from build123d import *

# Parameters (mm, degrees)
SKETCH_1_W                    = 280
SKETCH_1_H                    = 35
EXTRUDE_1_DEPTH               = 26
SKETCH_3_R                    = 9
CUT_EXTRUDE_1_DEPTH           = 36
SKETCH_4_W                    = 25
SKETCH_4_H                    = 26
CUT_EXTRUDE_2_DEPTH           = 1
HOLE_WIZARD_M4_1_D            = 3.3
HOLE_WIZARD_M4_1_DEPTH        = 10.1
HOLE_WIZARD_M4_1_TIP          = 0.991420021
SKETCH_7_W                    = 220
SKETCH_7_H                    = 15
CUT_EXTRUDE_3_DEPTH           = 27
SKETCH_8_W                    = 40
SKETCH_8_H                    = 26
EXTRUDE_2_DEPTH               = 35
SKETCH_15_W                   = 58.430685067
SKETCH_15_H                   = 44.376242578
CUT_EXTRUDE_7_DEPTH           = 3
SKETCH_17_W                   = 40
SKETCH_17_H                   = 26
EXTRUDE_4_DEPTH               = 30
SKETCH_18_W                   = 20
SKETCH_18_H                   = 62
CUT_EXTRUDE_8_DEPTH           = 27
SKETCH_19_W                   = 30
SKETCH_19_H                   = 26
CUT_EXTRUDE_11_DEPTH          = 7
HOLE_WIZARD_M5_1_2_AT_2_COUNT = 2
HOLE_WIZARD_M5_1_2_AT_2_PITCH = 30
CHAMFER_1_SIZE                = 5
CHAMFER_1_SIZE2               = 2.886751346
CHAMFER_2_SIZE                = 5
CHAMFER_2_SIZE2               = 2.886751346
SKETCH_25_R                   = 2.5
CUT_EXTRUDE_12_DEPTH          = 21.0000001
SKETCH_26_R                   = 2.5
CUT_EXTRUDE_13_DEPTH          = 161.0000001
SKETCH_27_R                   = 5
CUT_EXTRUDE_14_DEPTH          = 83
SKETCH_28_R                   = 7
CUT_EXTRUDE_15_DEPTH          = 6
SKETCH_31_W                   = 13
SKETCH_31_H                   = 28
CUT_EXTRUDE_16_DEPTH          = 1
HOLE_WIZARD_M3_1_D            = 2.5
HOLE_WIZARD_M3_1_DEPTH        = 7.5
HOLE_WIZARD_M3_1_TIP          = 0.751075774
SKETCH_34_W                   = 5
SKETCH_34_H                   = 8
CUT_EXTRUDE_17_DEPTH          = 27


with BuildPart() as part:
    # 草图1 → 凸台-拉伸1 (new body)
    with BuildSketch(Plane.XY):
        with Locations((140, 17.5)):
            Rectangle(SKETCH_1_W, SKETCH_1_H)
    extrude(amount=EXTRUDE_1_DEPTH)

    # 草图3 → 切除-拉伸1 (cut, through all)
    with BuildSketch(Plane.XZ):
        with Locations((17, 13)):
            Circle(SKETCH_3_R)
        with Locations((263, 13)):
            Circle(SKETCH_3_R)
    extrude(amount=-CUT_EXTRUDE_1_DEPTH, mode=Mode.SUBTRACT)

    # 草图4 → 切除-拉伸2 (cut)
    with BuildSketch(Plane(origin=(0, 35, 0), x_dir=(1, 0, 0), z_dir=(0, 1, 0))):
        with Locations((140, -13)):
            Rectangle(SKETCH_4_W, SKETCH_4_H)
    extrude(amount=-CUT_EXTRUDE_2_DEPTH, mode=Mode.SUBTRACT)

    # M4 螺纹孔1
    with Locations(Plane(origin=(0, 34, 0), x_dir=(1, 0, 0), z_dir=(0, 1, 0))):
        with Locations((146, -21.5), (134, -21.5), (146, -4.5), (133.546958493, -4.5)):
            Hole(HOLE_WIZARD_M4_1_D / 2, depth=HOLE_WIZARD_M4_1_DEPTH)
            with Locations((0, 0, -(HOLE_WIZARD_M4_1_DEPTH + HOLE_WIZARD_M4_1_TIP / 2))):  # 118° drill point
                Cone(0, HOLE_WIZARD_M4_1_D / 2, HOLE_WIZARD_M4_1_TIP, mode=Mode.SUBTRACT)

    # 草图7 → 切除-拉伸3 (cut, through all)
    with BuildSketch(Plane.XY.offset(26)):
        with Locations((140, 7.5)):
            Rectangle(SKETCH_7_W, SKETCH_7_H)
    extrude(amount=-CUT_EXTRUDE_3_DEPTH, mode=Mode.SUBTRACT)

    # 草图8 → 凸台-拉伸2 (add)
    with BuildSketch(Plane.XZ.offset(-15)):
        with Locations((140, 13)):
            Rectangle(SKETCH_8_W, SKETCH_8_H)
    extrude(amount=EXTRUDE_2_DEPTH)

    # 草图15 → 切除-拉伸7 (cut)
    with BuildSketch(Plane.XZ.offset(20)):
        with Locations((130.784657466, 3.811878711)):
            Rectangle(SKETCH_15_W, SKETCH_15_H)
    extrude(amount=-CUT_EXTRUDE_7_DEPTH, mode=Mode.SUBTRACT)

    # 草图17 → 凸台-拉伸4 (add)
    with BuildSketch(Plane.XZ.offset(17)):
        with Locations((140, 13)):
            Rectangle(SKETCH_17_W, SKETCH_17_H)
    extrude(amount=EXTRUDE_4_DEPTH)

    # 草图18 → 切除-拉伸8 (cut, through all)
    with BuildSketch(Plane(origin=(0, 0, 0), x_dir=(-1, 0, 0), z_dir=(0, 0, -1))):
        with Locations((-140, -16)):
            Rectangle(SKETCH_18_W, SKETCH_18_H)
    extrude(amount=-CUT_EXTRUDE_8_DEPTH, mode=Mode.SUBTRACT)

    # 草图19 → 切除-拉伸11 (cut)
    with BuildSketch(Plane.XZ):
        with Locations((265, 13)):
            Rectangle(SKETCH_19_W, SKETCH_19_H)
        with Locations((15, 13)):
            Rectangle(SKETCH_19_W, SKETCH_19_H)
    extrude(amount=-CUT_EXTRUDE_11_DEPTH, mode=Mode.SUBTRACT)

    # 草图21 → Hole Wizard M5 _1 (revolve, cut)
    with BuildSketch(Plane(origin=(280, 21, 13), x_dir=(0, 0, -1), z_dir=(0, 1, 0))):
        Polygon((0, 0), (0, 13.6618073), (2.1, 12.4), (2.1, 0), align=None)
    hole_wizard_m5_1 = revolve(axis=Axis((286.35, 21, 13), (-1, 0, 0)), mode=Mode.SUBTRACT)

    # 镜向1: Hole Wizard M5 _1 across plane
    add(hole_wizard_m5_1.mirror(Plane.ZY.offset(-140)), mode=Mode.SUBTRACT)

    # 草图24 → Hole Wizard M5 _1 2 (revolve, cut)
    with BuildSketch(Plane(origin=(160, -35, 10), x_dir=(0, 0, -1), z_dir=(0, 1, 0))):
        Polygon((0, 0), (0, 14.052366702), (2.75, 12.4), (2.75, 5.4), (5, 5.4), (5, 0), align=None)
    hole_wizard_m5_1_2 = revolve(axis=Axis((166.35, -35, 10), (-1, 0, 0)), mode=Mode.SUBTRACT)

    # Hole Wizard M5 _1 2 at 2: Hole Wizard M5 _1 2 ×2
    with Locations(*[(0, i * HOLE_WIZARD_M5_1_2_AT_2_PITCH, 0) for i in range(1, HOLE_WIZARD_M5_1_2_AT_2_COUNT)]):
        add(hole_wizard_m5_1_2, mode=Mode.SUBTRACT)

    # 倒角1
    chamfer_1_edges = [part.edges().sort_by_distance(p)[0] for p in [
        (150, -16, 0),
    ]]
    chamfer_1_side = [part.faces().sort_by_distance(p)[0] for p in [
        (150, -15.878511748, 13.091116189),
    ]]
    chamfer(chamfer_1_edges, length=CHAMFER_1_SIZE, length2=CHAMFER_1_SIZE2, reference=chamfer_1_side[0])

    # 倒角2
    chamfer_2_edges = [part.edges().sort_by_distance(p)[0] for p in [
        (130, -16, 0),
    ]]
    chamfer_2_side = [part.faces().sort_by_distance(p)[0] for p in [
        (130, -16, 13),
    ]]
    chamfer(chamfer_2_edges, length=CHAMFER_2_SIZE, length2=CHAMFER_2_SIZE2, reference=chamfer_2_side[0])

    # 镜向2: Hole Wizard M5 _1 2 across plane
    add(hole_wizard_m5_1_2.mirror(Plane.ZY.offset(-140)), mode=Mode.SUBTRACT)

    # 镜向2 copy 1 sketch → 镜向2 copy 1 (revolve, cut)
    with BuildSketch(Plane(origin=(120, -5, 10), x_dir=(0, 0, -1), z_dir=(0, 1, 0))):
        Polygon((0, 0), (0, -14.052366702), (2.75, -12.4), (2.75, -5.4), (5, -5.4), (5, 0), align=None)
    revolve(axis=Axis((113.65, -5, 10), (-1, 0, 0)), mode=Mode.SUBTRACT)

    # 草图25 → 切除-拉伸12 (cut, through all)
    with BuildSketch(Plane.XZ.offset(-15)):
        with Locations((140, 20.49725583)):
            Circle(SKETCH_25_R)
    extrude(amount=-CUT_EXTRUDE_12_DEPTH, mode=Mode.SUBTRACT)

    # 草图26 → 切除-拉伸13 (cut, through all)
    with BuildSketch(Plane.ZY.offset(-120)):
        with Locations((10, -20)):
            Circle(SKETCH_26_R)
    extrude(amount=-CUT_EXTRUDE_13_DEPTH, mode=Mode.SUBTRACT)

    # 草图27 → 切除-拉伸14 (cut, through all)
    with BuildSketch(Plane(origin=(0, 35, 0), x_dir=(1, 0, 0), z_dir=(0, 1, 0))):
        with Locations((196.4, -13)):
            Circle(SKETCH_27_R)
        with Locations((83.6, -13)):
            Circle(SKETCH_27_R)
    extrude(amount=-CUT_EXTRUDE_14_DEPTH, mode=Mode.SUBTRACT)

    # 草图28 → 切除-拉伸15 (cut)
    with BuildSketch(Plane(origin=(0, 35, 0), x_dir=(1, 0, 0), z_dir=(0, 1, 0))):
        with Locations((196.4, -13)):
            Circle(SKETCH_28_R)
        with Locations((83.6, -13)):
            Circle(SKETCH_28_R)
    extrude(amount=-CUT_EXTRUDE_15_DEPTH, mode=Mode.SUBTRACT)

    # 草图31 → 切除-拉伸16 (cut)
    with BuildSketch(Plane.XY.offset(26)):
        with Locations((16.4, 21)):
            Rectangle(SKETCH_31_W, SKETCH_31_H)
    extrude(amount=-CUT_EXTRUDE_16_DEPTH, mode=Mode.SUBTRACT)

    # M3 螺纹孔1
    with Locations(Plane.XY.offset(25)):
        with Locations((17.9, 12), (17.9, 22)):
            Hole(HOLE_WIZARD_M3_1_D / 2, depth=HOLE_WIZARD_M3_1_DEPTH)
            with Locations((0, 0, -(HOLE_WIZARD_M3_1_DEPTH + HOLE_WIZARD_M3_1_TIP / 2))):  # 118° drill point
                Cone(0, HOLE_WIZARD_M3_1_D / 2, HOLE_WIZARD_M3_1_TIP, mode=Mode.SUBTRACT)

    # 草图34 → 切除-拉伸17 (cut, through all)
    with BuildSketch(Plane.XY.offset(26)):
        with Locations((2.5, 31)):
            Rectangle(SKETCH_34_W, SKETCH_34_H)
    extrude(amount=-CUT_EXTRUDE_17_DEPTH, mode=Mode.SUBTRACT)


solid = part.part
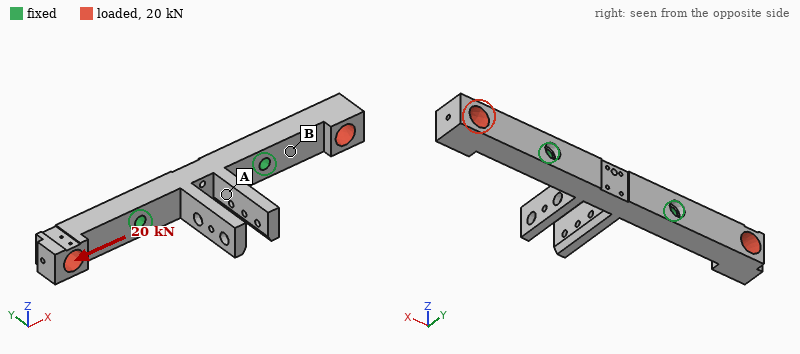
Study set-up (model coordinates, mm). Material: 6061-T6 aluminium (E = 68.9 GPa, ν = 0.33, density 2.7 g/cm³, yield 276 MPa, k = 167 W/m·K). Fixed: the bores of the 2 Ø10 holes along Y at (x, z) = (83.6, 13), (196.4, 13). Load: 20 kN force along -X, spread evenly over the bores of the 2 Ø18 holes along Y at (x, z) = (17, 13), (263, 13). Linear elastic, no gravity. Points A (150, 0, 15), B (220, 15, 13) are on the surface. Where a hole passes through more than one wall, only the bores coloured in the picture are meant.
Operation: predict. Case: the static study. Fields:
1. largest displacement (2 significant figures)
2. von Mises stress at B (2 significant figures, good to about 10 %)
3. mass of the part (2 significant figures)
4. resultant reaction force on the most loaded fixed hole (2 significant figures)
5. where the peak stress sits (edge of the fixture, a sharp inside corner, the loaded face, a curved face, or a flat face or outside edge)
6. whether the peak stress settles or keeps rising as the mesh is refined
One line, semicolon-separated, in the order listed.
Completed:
0.12 mm; 44 MPa; 450 g; 10 kN; a sharp inside corner; keeps rising
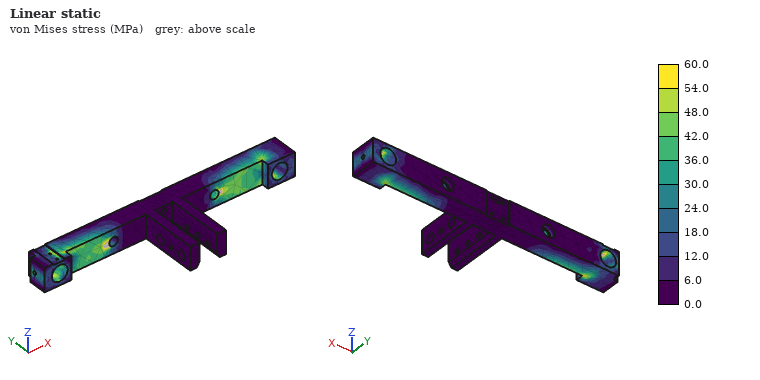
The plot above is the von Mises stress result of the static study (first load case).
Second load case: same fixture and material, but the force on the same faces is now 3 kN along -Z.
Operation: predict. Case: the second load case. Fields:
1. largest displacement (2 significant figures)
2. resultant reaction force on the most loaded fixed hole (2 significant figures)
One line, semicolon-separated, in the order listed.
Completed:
0.17 mm; 1.5 kN
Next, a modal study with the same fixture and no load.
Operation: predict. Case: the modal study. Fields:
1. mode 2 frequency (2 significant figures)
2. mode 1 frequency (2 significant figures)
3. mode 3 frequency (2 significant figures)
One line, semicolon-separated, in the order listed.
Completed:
1800 Hz; 1800 Hz; 2000 Hz
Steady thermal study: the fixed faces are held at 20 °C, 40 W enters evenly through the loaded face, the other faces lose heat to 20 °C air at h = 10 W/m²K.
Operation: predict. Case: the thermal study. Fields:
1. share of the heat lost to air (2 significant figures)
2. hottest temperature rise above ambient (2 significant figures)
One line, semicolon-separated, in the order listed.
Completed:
4.6 %; 18 K
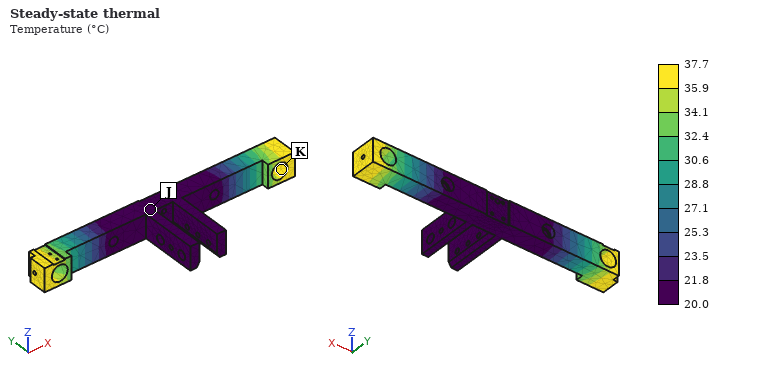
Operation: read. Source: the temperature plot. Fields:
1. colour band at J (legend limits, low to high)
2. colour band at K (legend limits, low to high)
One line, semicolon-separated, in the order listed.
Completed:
20.0 to 21.8 °C; 35.9 to 37.7 °C
